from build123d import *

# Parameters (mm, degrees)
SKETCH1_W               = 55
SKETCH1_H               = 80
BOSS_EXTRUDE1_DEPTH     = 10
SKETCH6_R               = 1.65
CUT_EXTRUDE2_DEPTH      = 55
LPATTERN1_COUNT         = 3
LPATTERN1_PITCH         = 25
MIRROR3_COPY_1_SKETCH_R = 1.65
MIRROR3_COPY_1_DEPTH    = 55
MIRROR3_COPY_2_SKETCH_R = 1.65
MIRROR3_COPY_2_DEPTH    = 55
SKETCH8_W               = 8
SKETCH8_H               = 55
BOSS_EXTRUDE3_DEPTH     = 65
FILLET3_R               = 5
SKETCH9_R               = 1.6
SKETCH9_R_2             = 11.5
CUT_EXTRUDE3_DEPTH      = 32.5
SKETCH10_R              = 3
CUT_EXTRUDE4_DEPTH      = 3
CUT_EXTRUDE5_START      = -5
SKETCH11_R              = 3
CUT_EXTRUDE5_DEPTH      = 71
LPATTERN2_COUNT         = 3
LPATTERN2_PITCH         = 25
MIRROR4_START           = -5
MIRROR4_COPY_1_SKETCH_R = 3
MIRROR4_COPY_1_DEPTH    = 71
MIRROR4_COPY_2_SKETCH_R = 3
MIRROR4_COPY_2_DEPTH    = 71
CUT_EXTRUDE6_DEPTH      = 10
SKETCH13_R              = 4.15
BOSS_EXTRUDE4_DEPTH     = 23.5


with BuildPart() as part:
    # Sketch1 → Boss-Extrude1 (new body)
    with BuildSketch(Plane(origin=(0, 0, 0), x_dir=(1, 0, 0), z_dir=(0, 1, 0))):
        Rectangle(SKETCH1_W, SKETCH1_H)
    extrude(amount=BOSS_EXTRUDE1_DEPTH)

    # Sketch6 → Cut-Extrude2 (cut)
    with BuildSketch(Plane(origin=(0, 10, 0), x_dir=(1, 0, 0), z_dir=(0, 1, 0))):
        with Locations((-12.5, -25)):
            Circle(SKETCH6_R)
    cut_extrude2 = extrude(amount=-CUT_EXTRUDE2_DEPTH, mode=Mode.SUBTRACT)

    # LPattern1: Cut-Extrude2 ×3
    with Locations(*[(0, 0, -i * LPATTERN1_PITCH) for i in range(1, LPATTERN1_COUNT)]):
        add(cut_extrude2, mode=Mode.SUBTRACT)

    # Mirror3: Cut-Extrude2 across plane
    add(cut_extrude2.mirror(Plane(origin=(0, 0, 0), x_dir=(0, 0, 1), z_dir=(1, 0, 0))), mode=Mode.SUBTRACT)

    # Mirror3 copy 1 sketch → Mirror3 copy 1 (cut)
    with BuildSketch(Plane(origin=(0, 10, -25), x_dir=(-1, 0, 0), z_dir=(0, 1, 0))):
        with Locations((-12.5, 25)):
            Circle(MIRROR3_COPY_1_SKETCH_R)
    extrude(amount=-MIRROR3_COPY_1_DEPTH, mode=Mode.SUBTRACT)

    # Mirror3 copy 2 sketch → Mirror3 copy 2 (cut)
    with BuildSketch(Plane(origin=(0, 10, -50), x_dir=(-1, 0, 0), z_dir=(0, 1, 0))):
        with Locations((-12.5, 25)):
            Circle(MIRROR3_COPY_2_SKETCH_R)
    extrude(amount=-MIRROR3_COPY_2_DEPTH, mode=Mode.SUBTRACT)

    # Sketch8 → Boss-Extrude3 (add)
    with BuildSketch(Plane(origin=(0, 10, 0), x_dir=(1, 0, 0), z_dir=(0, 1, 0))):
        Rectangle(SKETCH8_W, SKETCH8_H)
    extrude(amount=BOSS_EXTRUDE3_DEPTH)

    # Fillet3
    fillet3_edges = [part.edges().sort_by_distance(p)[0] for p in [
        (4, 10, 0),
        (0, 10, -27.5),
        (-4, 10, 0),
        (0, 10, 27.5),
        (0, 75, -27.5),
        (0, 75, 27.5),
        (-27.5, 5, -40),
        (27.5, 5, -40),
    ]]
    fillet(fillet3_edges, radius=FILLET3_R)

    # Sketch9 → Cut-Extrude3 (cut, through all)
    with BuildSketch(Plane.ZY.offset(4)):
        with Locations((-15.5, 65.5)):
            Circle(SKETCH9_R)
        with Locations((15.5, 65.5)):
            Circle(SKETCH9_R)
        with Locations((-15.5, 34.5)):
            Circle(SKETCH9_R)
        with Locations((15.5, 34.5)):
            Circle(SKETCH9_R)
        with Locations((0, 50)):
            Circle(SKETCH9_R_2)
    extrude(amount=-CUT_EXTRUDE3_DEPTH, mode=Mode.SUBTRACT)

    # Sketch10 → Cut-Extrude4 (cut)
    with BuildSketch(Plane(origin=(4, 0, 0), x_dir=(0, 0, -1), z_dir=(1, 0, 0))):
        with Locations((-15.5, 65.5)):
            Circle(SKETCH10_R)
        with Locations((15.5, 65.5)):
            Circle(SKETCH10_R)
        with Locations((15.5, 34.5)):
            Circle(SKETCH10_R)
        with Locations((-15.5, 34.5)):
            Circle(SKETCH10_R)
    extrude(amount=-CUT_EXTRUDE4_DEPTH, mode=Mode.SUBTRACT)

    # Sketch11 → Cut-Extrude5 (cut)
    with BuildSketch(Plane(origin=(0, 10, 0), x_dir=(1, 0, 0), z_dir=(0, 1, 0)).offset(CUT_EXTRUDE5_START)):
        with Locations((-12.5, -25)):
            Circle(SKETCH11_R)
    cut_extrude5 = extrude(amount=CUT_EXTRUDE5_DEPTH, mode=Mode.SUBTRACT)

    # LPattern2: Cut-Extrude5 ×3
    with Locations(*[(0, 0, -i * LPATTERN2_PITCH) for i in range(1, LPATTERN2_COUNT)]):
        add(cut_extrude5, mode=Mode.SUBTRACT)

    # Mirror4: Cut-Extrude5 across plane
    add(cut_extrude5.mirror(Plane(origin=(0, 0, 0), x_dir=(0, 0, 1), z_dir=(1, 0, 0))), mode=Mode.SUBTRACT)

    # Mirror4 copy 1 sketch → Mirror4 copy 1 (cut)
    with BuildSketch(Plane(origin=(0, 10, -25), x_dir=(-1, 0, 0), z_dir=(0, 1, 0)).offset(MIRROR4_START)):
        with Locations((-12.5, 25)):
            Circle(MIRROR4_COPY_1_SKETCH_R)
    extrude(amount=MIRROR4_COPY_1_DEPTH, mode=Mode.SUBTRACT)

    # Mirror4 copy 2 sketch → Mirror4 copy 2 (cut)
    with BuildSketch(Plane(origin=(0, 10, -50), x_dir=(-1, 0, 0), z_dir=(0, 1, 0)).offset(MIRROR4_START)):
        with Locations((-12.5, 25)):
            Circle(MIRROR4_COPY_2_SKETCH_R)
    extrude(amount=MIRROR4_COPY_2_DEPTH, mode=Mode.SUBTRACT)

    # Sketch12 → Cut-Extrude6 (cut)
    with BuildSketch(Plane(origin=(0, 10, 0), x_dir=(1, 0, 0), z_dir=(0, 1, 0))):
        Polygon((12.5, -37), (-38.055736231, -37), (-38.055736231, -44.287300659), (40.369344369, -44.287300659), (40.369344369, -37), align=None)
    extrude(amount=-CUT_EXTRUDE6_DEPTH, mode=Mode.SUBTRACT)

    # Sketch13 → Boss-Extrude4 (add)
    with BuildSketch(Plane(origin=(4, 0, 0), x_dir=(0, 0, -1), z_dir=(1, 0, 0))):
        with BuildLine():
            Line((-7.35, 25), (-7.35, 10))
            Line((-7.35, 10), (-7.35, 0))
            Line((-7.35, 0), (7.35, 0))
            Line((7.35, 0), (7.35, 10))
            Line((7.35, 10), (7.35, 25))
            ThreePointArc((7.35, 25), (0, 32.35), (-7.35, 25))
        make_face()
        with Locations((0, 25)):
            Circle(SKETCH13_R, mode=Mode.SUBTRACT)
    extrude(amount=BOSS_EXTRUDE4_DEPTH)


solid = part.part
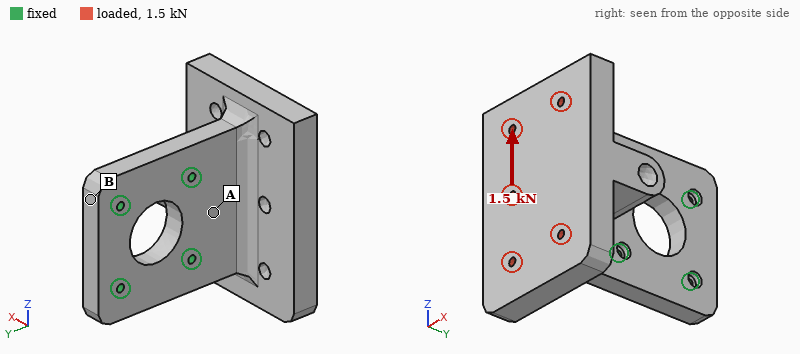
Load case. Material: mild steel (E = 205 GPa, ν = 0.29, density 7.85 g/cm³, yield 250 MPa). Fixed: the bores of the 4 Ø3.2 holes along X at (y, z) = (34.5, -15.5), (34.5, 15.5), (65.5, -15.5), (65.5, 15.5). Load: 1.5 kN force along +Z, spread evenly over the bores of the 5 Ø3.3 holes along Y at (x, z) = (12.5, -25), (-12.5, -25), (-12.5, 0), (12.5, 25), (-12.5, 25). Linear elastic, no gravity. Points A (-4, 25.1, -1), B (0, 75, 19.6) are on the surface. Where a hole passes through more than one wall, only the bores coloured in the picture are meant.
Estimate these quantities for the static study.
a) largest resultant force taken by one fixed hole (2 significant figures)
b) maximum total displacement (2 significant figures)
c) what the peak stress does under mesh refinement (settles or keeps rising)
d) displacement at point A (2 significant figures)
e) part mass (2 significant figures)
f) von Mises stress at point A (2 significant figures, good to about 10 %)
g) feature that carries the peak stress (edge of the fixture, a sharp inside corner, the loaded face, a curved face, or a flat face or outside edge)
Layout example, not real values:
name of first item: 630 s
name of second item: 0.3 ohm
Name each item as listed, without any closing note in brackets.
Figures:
largest resultant force taken by one fixed hole: 1.3 kN
maximum total displacement: 6.5 µm
what the peak stress does under mesh refinement: keeps rising
displacement at point A: 1.1 µm
part mass: 570 g
von Mises stress at point A: 11 MPa
feature that carries the peak stress: edge of the fixture
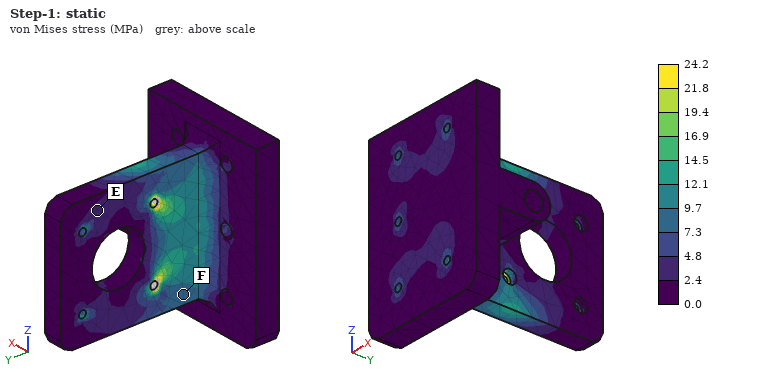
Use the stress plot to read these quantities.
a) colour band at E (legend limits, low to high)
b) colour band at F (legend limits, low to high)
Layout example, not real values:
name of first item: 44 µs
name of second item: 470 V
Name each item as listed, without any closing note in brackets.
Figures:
colour band at E: 2.4 to 4.8 MPa
colour band at F: 7.3 to 9.7 MPa
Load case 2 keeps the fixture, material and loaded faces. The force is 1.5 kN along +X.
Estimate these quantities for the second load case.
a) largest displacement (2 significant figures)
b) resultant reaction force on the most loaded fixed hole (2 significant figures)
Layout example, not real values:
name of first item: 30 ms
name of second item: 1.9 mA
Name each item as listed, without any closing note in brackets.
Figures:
largest displacement: 76 µm
resultant reaction force on the most loaded fixed hole: 1.4 kN
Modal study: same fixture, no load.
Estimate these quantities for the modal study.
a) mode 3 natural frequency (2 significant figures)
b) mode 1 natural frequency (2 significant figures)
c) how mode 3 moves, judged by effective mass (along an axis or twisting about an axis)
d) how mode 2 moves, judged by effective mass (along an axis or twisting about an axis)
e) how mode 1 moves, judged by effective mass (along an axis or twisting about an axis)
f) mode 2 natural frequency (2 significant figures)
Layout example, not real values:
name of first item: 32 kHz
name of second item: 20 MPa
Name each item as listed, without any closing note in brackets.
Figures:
mode 3 natural frequency: 5500 Hz
mode 1 natural frequency: 1300 Hz
how mode 3 moves, judged by effective mass: along Z
how mode 2 moves, judged by effective mass: twisting about Y
how mode 1 moves, judged by effective mass: along X
mode 2 natural frequency: 2800 Hz
